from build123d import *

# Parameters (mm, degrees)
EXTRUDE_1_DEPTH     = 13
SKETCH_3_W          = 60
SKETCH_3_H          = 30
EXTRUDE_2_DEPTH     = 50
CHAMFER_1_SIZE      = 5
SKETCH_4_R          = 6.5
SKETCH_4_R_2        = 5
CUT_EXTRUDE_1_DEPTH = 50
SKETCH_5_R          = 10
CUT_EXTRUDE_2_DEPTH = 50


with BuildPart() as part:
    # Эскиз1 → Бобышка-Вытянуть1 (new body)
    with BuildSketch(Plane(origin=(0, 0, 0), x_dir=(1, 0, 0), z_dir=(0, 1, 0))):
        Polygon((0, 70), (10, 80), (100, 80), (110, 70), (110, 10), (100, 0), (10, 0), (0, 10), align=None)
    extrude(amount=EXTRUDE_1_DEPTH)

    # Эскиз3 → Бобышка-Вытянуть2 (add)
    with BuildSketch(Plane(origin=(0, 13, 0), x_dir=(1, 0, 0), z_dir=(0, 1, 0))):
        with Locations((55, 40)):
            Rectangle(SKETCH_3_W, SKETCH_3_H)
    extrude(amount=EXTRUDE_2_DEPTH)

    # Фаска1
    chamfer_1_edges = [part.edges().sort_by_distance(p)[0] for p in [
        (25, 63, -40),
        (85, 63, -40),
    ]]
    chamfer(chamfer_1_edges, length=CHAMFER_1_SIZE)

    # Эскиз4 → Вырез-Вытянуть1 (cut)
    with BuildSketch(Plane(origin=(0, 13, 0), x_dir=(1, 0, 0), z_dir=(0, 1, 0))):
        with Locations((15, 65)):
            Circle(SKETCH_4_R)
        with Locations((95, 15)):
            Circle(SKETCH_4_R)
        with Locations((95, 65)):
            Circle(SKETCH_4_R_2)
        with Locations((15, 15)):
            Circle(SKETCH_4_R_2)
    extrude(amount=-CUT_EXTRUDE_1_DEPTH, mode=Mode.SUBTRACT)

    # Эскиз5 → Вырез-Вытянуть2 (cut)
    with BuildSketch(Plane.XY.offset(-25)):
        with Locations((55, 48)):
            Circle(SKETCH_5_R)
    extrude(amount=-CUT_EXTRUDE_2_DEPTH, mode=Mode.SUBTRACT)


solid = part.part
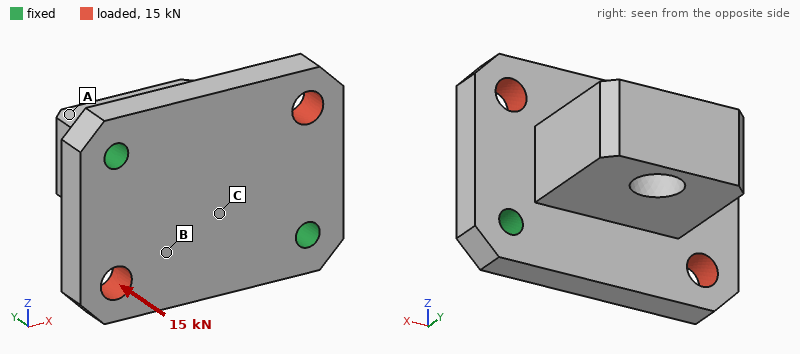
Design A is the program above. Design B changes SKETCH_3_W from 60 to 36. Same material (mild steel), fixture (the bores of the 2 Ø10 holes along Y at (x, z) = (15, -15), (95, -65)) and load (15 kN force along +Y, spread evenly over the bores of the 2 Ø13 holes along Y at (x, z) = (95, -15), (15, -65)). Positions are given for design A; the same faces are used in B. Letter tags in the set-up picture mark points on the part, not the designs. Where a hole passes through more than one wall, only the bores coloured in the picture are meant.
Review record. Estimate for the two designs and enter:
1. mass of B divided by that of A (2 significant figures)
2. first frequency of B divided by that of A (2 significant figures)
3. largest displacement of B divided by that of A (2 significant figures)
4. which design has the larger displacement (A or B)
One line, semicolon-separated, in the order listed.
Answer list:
0.81; 1.2; 1.4; B
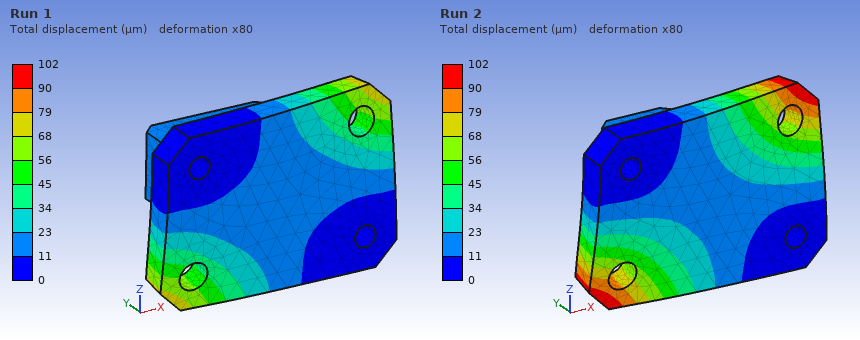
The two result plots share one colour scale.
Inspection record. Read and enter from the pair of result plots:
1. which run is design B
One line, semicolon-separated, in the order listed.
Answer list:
Run 2
